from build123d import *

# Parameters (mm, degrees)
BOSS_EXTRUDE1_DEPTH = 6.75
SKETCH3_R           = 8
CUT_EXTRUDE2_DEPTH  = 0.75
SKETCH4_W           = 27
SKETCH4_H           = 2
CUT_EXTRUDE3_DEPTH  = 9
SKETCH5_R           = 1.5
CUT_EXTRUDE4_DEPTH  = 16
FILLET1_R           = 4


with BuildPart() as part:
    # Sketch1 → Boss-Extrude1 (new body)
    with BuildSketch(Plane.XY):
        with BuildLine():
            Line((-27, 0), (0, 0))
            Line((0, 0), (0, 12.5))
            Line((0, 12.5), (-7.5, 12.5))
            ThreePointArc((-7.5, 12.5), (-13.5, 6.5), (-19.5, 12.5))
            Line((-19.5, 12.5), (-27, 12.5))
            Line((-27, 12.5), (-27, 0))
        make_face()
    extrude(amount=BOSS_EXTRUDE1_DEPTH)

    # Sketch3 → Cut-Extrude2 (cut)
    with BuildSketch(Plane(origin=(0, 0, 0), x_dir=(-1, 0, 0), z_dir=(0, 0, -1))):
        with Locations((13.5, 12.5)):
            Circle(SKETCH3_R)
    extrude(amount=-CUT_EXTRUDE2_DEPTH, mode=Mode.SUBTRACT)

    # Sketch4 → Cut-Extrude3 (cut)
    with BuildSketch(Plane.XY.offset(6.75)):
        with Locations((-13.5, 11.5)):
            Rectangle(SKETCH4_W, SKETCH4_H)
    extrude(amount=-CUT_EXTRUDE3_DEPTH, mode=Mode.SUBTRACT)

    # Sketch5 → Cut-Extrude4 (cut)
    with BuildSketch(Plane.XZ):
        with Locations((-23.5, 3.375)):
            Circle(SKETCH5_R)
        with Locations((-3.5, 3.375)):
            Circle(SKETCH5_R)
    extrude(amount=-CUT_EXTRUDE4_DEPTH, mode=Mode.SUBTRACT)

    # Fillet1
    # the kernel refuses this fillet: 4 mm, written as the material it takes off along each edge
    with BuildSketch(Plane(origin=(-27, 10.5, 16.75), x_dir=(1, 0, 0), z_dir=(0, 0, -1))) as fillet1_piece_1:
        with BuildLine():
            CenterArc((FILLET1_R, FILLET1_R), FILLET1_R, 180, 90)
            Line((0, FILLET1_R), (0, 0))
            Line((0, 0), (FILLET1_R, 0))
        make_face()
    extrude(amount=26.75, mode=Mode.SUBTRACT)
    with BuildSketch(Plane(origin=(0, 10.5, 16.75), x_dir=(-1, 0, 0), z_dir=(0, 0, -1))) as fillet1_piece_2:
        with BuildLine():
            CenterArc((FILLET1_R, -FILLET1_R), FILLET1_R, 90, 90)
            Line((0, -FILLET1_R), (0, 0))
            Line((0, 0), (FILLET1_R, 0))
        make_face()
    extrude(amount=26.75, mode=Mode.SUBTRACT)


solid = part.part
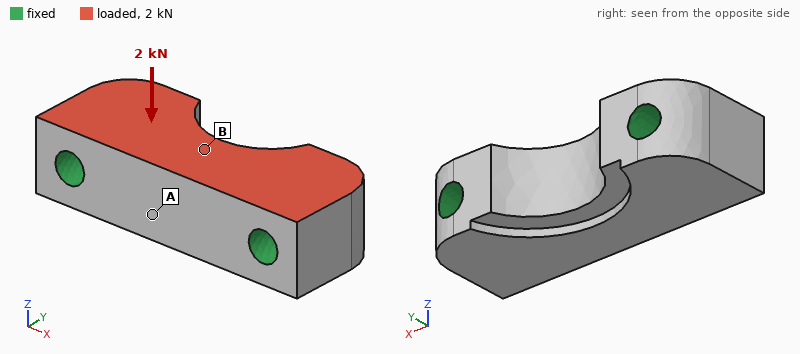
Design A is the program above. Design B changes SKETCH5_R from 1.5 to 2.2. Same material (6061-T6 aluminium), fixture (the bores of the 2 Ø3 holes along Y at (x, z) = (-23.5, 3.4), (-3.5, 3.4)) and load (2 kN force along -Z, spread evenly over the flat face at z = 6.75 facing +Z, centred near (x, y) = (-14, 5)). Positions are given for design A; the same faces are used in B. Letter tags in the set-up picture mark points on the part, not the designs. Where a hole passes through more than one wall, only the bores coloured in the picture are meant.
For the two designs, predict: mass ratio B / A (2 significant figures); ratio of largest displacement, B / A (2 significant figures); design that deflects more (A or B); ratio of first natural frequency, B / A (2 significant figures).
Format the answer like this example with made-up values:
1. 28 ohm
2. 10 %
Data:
1. 0.89
2. 0.75
3. A
4. 1.2
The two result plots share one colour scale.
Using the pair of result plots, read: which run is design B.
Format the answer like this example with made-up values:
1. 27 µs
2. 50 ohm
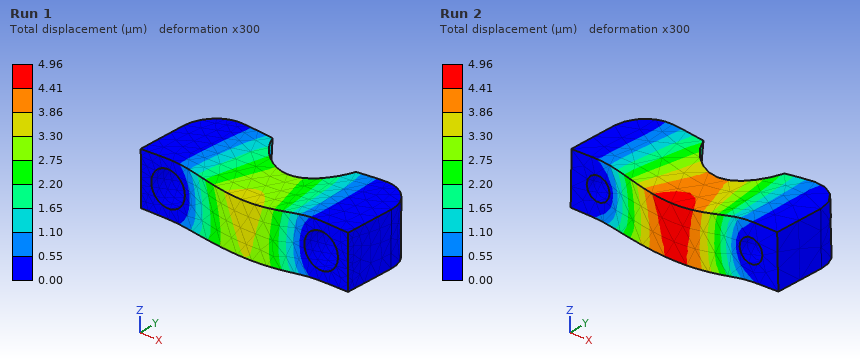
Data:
1. Run 1
